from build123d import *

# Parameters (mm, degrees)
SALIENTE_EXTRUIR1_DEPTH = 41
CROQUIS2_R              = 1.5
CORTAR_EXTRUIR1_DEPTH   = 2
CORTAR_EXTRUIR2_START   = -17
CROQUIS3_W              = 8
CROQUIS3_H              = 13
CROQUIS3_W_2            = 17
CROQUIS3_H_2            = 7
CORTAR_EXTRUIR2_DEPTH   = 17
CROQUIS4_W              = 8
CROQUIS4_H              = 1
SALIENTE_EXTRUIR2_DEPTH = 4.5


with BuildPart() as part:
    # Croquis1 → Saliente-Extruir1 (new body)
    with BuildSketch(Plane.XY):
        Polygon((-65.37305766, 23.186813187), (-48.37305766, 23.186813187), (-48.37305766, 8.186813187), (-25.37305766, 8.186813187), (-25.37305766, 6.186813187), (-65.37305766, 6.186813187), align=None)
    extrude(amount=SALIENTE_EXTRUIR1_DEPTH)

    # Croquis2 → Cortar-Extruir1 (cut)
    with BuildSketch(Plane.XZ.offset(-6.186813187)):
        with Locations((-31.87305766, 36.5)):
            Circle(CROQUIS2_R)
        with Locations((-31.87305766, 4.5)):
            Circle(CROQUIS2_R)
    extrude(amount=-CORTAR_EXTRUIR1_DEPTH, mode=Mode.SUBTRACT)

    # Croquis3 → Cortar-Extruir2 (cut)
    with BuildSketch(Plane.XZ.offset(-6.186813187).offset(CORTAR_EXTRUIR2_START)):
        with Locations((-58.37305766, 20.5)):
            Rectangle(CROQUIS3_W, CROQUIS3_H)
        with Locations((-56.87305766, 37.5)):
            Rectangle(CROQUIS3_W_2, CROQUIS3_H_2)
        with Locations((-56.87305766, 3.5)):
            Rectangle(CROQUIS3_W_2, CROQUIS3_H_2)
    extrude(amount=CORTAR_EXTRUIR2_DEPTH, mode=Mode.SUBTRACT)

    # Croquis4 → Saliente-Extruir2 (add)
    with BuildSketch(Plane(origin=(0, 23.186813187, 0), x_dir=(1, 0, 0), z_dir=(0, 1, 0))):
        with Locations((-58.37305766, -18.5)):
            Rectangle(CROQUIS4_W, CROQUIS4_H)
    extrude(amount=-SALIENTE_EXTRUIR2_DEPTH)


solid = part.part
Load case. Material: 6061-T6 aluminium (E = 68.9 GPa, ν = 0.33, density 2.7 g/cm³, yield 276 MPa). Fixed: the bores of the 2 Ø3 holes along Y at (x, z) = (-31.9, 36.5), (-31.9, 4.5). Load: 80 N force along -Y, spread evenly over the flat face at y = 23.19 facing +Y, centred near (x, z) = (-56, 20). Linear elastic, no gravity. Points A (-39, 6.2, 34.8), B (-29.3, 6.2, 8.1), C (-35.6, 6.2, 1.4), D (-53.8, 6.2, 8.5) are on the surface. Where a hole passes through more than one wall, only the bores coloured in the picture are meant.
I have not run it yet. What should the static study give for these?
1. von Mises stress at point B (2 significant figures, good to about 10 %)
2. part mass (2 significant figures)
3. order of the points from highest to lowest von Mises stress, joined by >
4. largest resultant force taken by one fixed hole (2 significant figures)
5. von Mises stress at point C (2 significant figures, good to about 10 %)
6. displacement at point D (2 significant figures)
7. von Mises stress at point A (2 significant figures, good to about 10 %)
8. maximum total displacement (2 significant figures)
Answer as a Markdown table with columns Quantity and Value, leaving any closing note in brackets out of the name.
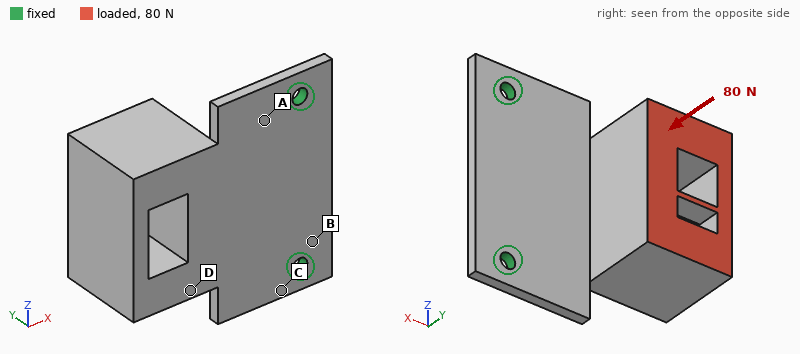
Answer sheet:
| Quantity | Value |
|---|---|
| von Mises stress at point B | 28 MPa |
| part mass | 21 g |
| order of the points from highest to lowest von Mises stress, joined by > | C > A > B > D |
| largest resultant force taken by one fixed hole | 40 N |
| von Mises stress at point C | 82 MPa |
| displacement at point D | 0.21 mm |
| von Mises stress at point A | 53 MPa |
| maximum total displacement | 0.43 mm |
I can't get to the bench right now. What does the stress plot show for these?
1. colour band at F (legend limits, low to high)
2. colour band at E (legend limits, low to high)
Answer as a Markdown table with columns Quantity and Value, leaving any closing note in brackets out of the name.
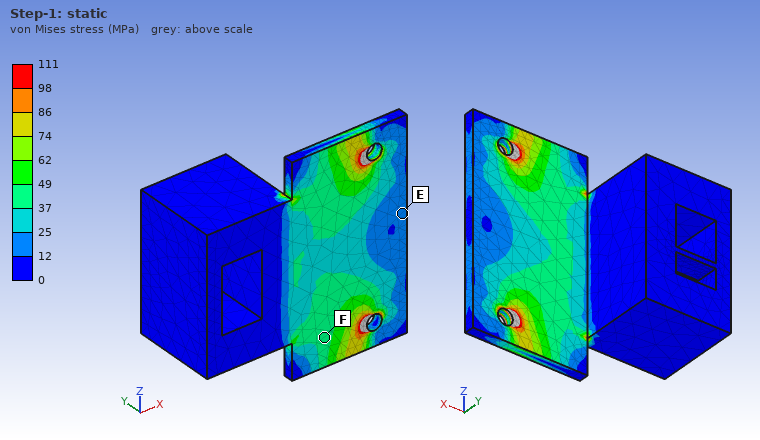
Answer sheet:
| Quantity | Value |
|---|---|
| colour band at F | 37 to 49 MPa |
| colour band at E | 12 to 25 MPa |
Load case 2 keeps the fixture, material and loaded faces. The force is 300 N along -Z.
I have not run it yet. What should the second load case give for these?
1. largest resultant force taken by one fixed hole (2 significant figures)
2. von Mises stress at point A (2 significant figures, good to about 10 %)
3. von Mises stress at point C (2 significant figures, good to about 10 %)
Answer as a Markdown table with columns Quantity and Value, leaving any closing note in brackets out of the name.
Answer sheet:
| Quantity | Value |
|---|---|
| largest resultant force taken by one fixed hole | 310 N |
| von Mises stress at point A | 57 MPa |
| von Mises stress at point C | 110 MPa |
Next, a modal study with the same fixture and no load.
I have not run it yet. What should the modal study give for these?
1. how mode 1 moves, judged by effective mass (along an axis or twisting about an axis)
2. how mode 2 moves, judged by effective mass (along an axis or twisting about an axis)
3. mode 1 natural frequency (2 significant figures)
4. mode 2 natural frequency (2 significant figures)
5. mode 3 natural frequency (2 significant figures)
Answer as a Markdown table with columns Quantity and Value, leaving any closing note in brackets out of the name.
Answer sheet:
| Quantity | Value |
|---|---|
| how mode 1 moves, judged by effective mass | along Y |
| how mode 2 moves, judged by effective mass | along Z |
| mode 1 natural frequency | 610 Hz |
| mode 2 natural frequency | 2200 Hz |
| mode 3 natural frequency | 3500 Hz |
